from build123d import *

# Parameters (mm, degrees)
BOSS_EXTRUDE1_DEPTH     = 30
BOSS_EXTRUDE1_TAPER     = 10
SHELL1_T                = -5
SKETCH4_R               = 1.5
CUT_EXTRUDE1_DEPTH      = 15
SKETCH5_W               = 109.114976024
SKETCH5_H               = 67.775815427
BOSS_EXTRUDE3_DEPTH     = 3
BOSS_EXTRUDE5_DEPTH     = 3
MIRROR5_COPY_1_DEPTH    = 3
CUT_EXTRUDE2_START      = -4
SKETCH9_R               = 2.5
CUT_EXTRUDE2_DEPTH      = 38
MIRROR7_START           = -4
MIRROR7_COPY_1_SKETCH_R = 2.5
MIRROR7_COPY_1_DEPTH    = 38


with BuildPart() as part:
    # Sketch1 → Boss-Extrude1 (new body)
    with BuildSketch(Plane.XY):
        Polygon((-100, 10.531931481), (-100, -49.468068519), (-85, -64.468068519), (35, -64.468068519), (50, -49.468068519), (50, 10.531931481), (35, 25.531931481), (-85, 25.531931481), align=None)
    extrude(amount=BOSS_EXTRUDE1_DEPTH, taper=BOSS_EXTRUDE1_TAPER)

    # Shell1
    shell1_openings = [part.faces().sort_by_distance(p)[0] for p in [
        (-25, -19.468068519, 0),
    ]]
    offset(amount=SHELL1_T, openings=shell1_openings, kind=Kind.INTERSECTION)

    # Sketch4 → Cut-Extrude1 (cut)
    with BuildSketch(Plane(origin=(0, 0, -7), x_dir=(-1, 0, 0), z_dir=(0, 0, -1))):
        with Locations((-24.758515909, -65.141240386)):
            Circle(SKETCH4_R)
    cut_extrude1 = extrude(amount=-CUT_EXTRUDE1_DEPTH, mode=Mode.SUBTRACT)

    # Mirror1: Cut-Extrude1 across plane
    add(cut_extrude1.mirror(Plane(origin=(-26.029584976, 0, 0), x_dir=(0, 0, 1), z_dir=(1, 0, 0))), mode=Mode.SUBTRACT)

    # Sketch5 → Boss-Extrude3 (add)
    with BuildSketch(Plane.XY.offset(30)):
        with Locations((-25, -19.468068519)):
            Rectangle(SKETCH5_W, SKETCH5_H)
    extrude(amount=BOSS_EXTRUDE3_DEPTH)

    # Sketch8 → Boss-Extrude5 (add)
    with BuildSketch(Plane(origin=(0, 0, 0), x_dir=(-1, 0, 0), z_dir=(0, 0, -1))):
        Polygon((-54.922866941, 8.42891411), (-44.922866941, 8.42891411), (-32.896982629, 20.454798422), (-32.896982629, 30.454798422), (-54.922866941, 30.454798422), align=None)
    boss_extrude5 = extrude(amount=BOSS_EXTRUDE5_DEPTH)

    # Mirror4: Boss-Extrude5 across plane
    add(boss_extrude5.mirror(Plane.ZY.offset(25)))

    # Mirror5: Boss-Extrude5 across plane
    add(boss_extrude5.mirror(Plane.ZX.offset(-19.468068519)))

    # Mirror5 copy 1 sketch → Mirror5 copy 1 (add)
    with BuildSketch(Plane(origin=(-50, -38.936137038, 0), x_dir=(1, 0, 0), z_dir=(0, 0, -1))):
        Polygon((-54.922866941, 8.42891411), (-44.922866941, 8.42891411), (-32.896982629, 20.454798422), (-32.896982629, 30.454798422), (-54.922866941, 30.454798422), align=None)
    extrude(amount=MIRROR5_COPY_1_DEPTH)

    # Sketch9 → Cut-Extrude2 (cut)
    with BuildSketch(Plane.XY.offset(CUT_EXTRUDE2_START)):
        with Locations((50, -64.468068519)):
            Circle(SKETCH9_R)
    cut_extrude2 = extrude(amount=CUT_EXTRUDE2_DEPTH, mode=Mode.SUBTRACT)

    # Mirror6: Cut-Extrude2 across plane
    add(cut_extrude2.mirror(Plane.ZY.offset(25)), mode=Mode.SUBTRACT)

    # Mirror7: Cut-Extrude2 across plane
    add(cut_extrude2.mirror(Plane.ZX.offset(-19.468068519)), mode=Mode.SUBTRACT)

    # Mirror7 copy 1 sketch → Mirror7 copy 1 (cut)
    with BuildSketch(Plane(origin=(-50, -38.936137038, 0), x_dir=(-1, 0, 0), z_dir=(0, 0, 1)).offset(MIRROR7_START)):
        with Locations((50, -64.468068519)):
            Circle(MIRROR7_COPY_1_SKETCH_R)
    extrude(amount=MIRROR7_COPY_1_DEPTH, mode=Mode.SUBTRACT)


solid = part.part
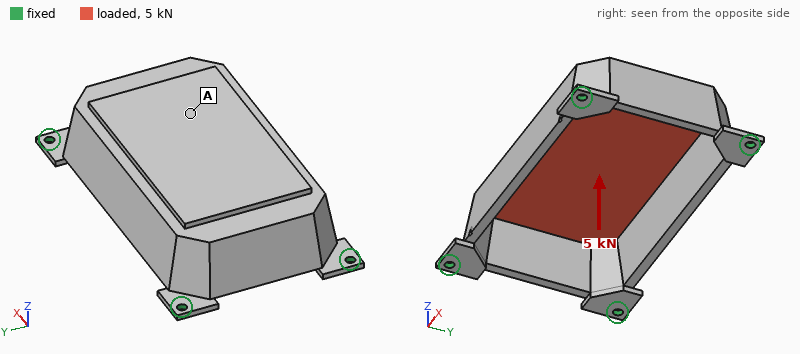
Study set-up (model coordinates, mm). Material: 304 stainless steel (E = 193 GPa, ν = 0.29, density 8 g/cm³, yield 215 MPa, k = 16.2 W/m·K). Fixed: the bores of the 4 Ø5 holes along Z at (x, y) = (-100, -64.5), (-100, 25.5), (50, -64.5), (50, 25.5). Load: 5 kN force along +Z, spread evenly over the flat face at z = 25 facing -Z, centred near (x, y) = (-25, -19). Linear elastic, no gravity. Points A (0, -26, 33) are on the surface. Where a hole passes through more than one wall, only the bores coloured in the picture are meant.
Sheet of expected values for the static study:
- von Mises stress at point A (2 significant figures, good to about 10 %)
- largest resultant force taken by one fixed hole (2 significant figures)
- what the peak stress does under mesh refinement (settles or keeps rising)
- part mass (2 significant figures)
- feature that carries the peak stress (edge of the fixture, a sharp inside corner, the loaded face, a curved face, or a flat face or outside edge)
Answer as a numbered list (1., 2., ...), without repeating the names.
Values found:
1. 19 MPa
2. 1.8 kN
3. keeps rising
4. 1.1 kg
5. edge of the fixture
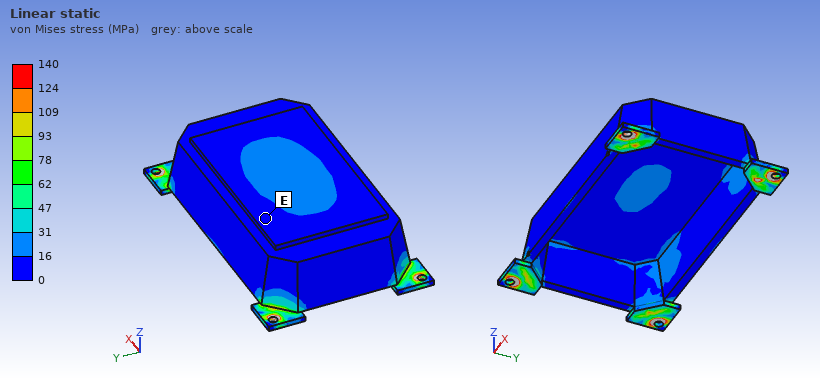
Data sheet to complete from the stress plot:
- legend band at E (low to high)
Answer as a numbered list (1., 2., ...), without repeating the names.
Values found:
1. 0 to 16 MPa
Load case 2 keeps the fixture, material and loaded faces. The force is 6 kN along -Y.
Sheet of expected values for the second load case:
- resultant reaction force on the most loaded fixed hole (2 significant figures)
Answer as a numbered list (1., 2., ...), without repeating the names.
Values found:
1. 1.8 kN
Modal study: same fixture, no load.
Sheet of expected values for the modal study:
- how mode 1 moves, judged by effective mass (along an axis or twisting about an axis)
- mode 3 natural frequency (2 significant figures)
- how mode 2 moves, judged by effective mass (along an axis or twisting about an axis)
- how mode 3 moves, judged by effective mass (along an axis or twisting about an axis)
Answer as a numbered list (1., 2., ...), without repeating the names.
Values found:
1. along Z
2. 3000 Hz
3. along Y
4. along X
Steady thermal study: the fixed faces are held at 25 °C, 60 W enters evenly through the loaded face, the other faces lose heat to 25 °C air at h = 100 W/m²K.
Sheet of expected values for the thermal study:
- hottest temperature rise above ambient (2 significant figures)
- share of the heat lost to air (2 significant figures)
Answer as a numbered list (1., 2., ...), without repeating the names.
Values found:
1. 38 K
2. 98 %
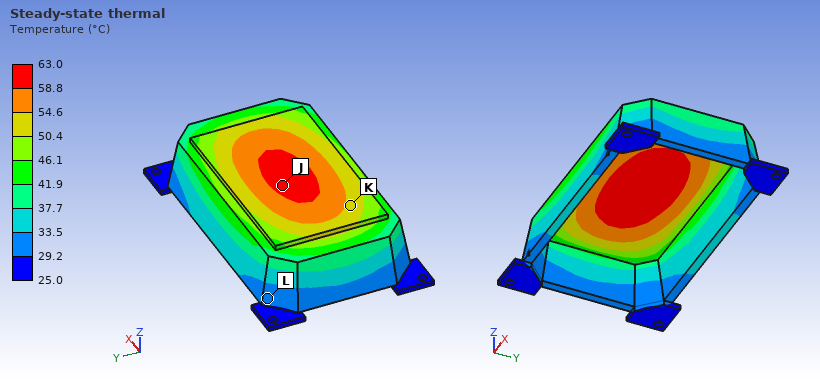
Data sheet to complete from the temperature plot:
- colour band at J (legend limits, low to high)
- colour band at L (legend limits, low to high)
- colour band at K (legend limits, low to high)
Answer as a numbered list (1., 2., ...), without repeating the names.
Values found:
1. 58.8 to 63.0 °C
2. 29.2 to 33.5 °C
3. 50.4 to 54.6 °C
